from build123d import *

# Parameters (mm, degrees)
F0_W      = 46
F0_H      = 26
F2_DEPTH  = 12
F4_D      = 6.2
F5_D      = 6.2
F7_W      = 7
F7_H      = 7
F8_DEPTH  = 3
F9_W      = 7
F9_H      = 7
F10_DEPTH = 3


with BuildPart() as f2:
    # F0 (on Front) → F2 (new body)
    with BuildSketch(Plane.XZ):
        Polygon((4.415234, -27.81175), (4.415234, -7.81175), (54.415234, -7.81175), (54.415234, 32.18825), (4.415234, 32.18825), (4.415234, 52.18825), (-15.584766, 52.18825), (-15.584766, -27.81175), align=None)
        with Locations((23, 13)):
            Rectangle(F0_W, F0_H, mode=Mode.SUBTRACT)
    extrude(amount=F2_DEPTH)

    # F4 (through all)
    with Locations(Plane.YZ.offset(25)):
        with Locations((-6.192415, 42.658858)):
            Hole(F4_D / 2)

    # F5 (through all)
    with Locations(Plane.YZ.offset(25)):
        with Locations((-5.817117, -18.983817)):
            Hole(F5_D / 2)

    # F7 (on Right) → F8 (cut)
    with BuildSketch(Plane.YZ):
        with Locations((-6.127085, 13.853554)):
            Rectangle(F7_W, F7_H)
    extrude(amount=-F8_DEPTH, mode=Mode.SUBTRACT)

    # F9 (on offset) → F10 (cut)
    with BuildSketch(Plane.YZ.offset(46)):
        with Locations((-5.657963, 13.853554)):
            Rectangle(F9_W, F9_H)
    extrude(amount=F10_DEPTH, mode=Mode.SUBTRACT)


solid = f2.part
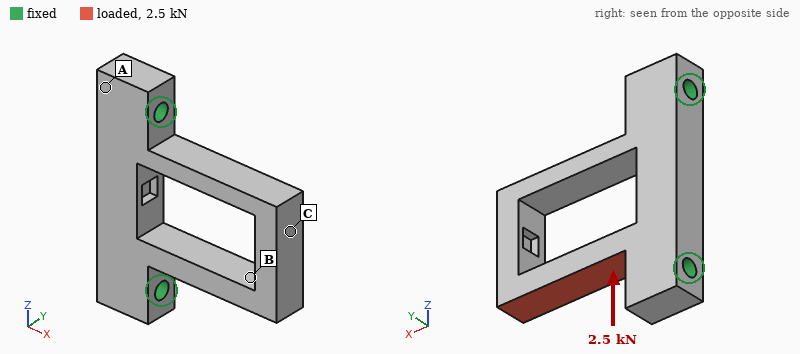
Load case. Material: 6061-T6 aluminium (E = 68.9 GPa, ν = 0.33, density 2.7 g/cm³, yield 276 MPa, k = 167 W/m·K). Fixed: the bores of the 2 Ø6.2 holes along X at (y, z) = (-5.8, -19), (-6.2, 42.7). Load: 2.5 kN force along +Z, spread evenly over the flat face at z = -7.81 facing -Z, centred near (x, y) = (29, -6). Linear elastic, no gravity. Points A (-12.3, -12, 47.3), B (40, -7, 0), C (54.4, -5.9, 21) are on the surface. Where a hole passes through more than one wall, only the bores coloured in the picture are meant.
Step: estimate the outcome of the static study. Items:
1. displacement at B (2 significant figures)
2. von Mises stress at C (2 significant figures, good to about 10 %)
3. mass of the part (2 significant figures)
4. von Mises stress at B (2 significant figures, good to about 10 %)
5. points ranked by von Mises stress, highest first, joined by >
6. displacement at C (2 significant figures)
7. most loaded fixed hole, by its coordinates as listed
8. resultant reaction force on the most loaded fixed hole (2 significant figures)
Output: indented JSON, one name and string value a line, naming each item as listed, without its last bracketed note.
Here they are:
{
  "displacement at B": "0.31 mm",
  "von Mises stress at C": "45 MPa",
  "mass of the part": "74 g",
  "von Mises stress at B": "110 MPa",
  "points ranked by von Mises stress, highest first, joined by >": "B > C > A",
  "displacement at C": "0.34 mm",
  "most loaded fixed hole, by its coordinates as listed": "(-5.8, -19)",
  "resultant reaction force on the most loaded fixed hole": "2.4 kN"
}
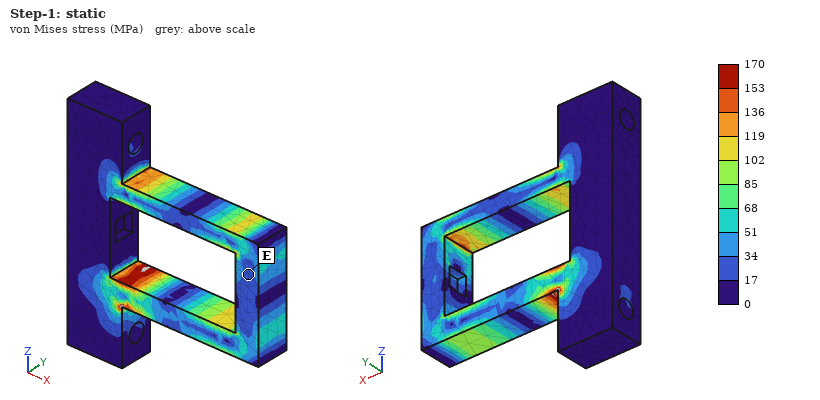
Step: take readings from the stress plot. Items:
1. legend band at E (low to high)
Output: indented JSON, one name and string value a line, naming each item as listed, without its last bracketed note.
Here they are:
{
  "legend band at E": "17 to 34 MPa"
}
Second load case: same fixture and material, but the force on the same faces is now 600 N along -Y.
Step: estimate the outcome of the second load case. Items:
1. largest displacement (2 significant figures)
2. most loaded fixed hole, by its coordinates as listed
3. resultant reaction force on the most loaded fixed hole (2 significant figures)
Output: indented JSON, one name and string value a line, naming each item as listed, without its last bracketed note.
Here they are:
{
  "largest displacement": "0.20 mm",
  "most loaded fixed hole, by its coordinates as listed": "(-5.8, -19)",
  "resultant reaction force on the most loaded fixed hole": "560 N"
}
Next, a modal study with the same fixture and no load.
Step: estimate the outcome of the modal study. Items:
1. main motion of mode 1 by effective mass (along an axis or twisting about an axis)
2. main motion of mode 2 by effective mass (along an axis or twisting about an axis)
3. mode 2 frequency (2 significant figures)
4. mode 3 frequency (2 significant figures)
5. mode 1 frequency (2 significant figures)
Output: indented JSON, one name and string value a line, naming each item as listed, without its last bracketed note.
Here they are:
{
  "main motion of mode 1 by effective mass": "along Y",
  "main motion of mode 2 by effective mass": "along Z",
  "mode 2 frequency": "2500 Hz",
  "mode 3 frequency": "4300 Hz",
  "mode 1 frequency": "2000 Hz"
}
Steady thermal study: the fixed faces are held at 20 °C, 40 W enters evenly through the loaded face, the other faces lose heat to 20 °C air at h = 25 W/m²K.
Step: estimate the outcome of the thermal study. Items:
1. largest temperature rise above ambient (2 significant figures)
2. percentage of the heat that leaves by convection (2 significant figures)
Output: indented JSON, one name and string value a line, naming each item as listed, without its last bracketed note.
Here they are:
{
  "largest temperature rise above ambient": "51 K",
  "percentage of the heat that leaves by convection": "9.5 %"
}
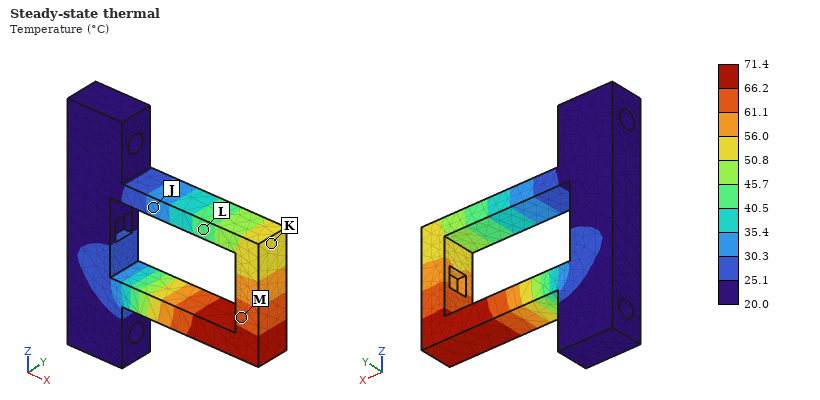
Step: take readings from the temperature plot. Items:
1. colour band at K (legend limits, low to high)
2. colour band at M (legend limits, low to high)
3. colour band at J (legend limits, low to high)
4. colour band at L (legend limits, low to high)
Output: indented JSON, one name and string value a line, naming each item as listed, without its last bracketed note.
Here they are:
{
  "colour band at K": "50.8 to 56.0 °C",
  "colour band at M": "61.1 to 66.2 °C",
  "colour band at J": "30.3 to 35.4 °C",
  "colour band at L": "40.5 to 45.7 °C"
}
